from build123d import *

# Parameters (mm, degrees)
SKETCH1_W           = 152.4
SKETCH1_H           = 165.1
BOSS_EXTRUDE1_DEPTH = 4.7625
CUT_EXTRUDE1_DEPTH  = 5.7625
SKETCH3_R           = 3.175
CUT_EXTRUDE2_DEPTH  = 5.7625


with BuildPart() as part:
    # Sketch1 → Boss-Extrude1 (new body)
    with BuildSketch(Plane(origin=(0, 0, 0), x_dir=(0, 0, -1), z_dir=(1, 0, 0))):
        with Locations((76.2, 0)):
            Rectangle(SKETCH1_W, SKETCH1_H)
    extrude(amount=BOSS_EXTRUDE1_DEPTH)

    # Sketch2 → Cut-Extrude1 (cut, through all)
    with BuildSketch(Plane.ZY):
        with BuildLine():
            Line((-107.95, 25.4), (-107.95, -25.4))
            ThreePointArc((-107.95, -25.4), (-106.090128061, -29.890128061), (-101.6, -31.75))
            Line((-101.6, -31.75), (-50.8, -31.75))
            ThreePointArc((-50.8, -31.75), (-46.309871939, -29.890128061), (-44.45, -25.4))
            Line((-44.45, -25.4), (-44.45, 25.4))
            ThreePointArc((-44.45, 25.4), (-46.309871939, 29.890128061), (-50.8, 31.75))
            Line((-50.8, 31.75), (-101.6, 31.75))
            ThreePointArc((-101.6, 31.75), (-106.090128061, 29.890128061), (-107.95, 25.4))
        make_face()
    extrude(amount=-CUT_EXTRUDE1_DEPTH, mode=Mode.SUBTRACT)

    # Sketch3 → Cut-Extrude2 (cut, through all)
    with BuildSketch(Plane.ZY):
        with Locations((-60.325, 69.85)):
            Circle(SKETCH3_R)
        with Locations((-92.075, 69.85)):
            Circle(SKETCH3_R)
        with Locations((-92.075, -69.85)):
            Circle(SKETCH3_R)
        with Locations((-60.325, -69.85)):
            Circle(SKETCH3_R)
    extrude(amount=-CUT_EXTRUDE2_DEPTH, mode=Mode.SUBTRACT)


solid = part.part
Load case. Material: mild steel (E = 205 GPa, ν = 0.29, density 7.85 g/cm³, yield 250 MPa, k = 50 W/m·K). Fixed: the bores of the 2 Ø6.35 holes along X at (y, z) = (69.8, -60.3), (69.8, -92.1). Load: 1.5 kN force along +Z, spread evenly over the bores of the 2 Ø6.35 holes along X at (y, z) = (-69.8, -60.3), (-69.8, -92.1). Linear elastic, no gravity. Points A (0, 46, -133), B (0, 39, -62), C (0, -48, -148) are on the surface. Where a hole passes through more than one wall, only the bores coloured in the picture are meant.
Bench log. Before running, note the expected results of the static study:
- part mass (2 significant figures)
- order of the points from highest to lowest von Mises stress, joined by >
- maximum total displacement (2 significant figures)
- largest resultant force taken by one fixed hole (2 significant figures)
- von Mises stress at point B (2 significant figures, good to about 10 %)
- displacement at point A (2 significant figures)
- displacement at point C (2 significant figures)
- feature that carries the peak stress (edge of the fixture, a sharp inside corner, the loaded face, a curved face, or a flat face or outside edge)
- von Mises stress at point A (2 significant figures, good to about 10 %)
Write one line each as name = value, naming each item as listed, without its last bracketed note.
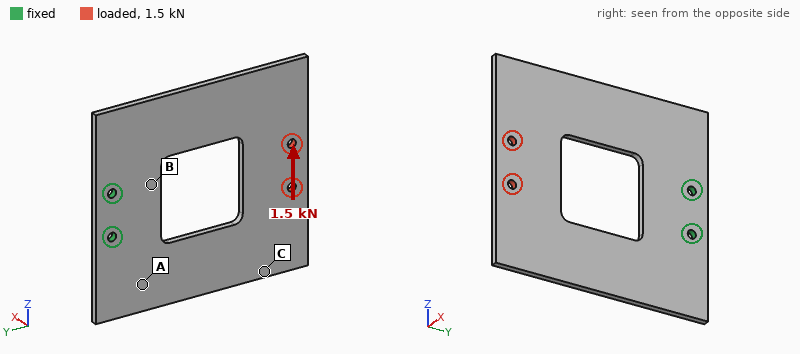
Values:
part mass = 790 g
order of the points from highest to lowest von Mises stress, joined by > = B > A > C
maximum total displacement = 0.10 mm
largest resultant force taken by one fixed hole = 5.6 kN
von Mises stress at point B = 26 MPa
displacement at point A = 0.029 mm
displacement at point C = 0.085 mm
feature that carries the peak stress = edge of the fixture
von Mises stress at point A = 12 MPa
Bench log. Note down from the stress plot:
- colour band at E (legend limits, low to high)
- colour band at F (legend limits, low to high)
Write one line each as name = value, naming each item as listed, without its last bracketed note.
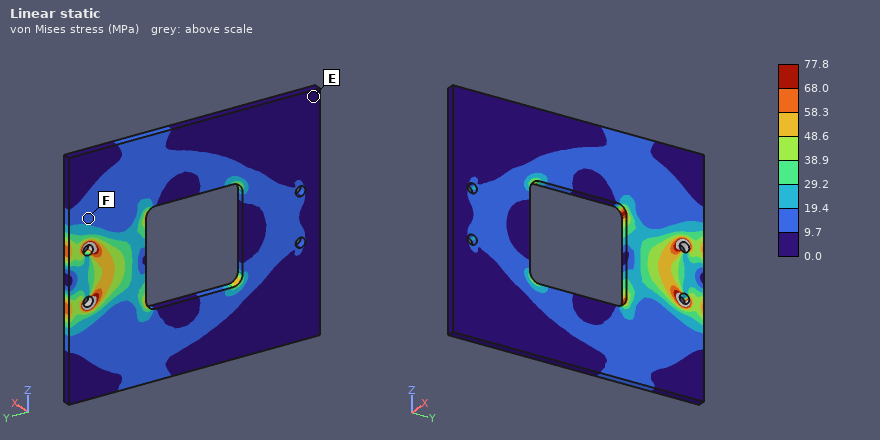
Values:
colour band at E = 0.0 to 9.7 MPa
colour band at F = 9.7 to 19.4 MPa
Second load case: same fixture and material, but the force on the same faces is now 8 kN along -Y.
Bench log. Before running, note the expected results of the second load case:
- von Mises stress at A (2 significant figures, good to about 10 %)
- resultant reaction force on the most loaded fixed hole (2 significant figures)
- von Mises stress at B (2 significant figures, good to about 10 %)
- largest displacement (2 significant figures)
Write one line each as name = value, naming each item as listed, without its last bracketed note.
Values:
von Mises stress at A = 12 MPa
resultant reaction force on the most loaded fixed hole = 4.4 kN
von Mises stress at B = 33 MPa
largest displacement = 41 µm
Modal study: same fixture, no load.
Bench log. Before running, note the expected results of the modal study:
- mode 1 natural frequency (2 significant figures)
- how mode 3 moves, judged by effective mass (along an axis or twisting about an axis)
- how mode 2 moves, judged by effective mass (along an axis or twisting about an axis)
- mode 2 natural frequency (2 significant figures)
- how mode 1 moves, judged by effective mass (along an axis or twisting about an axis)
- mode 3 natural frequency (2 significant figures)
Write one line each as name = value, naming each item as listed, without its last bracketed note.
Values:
mode 1 natural frequency = 130 Hz
how mode 3 moves, judged by effective mass = along X
how mode 2 moves, judged by effective mass = twisting about Y
mode 2 natural frequency = 280 Hz
how mode 1 moves, judged by effective mass = along X
mode 3 natural frequency = 710 Hz
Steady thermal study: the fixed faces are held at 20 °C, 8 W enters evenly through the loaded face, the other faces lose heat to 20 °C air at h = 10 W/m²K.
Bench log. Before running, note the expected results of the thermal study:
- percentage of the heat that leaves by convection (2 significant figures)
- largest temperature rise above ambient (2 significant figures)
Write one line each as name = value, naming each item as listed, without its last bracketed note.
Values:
percentage of the heat that leaves by convection = 71 %
largest temperature rise above ambient = 33 K
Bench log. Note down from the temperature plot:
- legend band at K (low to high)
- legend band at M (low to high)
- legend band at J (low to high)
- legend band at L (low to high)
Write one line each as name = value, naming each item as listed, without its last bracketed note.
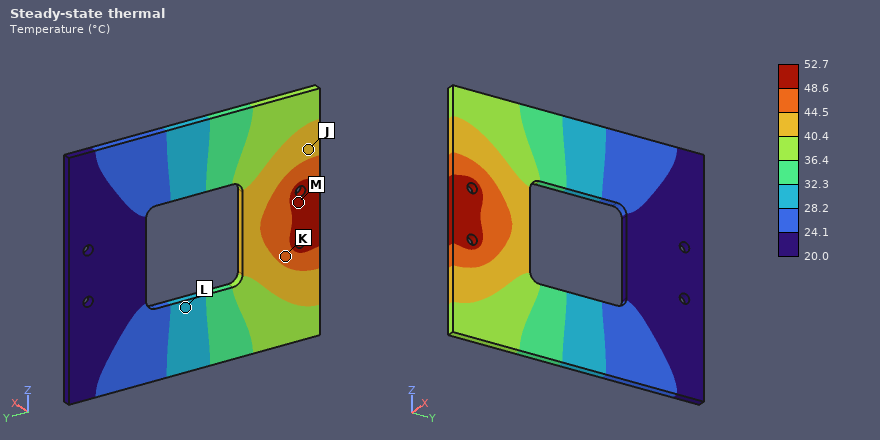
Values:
legend band at K = 44.5 to 48.6 °C
legend band at M = 48.6 to 52.7 °C
legend band at J = 40.4 to 44.5 °C
legend band at L = 28.2 to 32.3 °C
